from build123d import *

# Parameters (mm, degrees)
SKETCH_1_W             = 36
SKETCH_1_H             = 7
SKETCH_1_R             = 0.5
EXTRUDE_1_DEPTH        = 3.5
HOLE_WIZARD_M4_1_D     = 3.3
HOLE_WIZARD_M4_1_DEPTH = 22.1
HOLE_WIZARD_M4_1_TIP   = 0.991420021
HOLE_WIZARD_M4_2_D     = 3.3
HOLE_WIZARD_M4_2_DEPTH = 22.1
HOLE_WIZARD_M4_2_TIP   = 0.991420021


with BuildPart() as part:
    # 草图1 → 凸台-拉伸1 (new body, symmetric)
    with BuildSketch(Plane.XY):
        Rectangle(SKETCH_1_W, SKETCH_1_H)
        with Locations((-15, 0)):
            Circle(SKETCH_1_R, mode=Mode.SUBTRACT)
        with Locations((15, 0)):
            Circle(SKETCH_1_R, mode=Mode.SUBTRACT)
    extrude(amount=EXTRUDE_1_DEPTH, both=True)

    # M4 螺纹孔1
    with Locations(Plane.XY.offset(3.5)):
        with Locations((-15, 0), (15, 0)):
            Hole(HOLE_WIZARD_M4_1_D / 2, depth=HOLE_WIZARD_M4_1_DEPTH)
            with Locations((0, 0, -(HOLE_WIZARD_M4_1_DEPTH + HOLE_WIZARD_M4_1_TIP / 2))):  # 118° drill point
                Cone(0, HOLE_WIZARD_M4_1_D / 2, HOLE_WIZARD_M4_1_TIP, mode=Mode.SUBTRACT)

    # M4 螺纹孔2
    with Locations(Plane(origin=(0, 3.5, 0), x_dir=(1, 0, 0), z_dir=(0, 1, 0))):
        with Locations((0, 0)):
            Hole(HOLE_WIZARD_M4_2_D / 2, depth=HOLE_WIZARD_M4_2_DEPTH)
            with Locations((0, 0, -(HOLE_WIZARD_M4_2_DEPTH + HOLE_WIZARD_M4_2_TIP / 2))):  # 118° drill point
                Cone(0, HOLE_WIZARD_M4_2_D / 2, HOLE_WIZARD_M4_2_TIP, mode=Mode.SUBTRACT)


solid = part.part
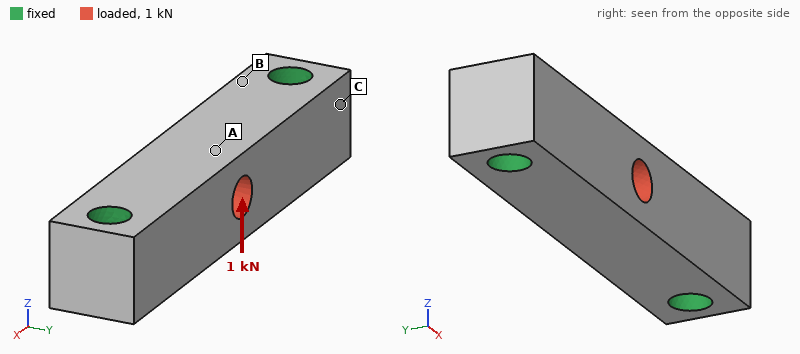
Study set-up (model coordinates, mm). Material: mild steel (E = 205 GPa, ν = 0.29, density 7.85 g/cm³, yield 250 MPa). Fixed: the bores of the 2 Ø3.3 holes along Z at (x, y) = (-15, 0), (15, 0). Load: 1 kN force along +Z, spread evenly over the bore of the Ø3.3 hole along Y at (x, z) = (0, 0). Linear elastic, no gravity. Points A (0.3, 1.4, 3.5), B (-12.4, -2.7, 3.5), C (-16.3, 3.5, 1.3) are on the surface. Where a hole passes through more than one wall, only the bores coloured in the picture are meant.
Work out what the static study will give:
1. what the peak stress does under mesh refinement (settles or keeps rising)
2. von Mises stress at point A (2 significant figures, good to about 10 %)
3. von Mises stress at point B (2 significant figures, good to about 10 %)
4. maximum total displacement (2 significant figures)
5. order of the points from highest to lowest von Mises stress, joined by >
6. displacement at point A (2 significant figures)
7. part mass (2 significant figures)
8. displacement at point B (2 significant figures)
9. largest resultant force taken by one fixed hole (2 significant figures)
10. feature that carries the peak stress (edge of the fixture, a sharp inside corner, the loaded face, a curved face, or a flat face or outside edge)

keeps rising
64 MPa
35 MPa
5.0 µm
A > B > C
4.7 µm
12 g
0.76 µm
500 N
edge of the fixture
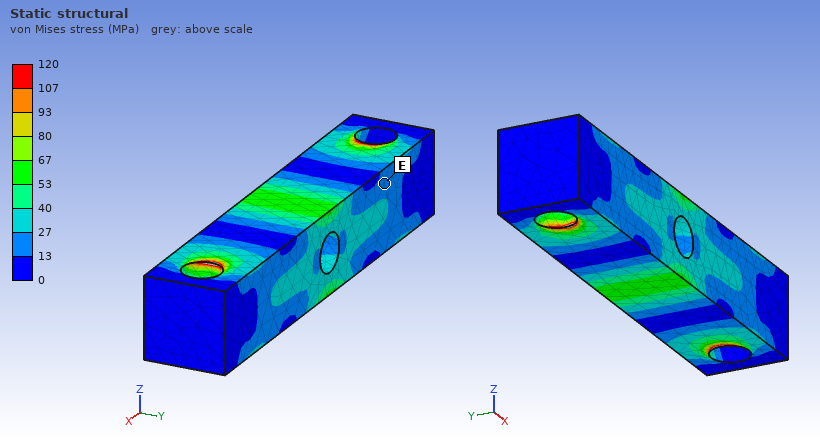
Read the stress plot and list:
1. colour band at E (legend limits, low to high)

13 to 27 MPa
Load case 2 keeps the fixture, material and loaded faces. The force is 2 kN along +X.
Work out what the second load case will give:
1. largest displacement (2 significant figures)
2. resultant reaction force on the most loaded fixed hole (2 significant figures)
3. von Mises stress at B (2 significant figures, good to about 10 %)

1.5 µm
1.0 kN
14 MPa
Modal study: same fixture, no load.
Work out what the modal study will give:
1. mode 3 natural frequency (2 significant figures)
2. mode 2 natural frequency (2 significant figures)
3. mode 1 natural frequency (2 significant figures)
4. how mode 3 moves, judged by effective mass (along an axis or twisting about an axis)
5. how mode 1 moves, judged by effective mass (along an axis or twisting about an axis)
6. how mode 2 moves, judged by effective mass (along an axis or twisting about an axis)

53 kHz
36 kHz
31 kHz
twisting about X
along Y
along Z
